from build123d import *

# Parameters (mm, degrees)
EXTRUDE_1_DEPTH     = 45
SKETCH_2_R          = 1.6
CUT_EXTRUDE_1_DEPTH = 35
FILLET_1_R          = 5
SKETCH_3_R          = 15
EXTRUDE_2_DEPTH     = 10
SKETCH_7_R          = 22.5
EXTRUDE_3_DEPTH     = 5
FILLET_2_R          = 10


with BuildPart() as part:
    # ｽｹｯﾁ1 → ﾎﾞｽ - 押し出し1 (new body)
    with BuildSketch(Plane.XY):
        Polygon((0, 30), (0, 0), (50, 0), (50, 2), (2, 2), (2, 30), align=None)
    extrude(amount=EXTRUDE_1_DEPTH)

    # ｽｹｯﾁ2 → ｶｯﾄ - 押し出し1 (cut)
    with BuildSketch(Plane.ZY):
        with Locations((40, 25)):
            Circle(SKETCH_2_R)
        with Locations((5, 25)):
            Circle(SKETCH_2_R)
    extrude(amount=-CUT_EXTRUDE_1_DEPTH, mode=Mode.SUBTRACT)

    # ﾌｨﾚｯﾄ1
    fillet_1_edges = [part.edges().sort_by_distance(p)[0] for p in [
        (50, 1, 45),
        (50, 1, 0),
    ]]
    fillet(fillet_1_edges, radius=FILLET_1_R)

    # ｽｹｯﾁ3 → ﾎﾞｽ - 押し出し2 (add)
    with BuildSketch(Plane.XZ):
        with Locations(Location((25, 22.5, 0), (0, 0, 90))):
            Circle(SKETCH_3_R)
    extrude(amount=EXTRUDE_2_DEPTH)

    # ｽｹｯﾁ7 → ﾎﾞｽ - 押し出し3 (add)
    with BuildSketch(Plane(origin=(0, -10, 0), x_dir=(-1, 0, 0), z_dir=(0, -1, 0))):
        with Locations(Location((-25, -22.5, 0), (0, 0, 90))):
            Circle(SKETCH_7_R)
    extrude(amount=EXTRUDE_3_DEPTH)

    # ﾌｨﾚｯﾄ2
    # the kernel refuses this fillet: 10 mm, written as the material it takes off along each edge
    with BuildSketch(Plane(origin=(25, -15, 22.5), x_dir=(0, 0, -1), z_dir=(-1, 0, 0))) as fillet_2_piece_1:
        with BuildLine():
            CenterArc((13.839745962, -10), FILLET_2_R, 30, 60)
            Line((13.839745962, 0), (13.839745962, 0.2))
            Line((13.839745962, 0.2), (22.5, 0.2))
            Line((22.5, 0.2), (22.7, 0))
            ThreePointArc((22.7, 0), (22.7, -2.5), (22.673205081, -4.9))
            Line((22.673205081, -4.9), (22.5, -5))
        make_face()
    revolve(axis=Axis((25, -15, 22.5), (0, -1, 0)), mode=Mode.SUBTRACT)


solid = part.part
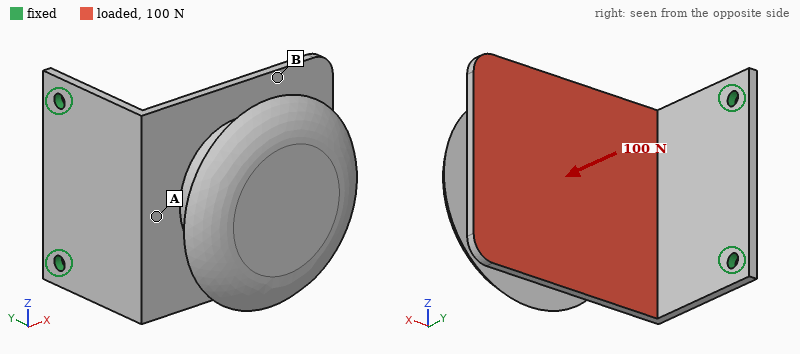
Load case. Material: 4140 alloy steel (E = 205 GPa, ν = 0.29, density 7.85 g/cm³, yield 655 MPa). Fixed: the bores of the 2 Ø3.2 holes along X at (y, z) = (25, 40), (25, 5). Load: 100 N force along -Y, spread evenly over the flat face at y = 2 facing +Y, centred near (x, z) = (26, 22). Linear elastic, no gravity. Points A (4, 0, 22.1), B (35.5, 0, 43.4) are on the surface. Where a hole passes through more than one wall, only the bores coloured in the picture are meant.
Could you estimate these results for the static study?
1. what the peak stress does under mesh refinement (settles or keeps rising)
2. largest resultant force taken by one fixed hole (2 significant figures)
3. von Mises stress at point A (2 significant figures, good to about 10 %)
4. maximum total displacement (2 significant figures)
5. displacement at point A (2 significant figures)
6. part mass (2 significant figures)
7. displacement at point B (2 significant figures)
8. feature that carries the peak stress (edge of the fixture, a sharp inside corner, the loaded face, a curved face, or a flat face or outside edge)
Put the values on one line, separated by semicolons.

keeps rising; 52 N; 68 MPa; 0.66 mm; 0.15 mm; 160 g; 0.46 mm; edge of the fixture
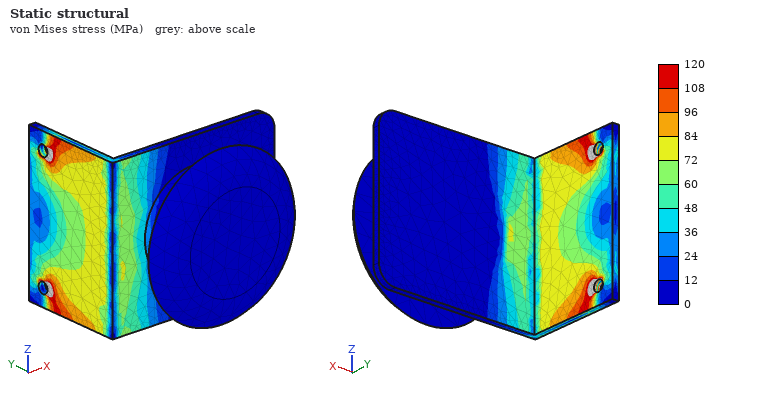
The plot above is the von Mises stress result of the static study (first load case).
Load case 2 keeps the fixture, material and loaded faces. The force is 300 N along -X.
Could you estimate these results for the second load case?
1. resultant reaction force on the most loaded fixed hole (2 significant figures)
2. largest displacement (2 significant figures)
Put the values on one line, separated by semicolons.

150 N; 0.78 mm
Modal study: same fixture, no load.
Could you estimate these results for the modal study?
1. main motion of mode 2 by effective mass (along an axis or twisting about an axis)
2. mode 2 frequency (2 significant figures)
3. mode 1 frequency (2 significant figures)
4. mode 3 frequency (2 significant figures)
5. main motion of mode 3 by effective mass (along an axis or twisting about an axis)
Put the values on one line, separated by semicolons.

along Z; 490 Hz; 180 Hz; 870 Hz; along X
